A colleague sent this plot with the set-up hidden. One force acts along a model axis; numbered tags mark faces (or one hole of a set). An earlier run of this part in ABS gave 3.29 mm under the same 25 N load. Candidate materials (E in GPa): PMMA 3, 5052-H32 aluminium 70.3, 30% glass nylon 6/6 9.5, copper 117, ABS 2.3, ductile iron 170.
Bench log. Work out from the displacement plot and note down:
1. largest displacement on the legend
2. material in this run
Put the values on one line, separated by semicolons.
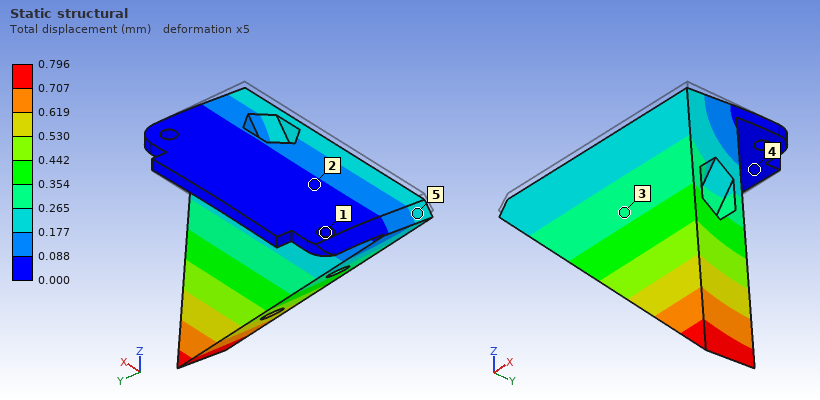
0.796 mm; 30% glass nylon 6/6
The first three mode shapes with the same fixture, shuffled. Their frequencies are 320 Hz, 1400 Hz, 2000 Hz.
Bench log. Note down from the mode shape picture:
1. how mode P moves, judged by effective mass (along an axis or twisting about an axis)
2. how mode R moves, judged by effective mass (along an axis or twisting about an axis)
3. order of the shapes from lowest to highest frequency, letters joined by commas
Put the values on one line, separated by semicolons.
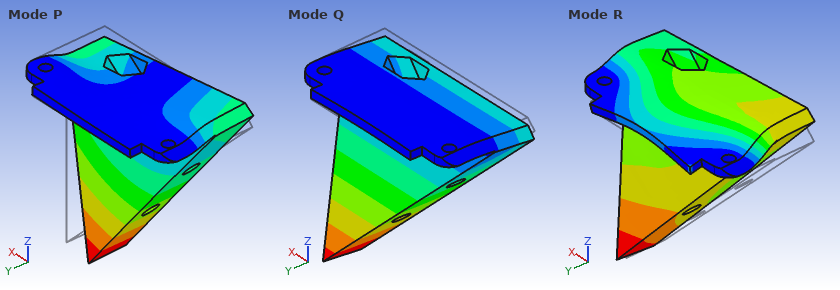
along X; along Z; Q, P, R
